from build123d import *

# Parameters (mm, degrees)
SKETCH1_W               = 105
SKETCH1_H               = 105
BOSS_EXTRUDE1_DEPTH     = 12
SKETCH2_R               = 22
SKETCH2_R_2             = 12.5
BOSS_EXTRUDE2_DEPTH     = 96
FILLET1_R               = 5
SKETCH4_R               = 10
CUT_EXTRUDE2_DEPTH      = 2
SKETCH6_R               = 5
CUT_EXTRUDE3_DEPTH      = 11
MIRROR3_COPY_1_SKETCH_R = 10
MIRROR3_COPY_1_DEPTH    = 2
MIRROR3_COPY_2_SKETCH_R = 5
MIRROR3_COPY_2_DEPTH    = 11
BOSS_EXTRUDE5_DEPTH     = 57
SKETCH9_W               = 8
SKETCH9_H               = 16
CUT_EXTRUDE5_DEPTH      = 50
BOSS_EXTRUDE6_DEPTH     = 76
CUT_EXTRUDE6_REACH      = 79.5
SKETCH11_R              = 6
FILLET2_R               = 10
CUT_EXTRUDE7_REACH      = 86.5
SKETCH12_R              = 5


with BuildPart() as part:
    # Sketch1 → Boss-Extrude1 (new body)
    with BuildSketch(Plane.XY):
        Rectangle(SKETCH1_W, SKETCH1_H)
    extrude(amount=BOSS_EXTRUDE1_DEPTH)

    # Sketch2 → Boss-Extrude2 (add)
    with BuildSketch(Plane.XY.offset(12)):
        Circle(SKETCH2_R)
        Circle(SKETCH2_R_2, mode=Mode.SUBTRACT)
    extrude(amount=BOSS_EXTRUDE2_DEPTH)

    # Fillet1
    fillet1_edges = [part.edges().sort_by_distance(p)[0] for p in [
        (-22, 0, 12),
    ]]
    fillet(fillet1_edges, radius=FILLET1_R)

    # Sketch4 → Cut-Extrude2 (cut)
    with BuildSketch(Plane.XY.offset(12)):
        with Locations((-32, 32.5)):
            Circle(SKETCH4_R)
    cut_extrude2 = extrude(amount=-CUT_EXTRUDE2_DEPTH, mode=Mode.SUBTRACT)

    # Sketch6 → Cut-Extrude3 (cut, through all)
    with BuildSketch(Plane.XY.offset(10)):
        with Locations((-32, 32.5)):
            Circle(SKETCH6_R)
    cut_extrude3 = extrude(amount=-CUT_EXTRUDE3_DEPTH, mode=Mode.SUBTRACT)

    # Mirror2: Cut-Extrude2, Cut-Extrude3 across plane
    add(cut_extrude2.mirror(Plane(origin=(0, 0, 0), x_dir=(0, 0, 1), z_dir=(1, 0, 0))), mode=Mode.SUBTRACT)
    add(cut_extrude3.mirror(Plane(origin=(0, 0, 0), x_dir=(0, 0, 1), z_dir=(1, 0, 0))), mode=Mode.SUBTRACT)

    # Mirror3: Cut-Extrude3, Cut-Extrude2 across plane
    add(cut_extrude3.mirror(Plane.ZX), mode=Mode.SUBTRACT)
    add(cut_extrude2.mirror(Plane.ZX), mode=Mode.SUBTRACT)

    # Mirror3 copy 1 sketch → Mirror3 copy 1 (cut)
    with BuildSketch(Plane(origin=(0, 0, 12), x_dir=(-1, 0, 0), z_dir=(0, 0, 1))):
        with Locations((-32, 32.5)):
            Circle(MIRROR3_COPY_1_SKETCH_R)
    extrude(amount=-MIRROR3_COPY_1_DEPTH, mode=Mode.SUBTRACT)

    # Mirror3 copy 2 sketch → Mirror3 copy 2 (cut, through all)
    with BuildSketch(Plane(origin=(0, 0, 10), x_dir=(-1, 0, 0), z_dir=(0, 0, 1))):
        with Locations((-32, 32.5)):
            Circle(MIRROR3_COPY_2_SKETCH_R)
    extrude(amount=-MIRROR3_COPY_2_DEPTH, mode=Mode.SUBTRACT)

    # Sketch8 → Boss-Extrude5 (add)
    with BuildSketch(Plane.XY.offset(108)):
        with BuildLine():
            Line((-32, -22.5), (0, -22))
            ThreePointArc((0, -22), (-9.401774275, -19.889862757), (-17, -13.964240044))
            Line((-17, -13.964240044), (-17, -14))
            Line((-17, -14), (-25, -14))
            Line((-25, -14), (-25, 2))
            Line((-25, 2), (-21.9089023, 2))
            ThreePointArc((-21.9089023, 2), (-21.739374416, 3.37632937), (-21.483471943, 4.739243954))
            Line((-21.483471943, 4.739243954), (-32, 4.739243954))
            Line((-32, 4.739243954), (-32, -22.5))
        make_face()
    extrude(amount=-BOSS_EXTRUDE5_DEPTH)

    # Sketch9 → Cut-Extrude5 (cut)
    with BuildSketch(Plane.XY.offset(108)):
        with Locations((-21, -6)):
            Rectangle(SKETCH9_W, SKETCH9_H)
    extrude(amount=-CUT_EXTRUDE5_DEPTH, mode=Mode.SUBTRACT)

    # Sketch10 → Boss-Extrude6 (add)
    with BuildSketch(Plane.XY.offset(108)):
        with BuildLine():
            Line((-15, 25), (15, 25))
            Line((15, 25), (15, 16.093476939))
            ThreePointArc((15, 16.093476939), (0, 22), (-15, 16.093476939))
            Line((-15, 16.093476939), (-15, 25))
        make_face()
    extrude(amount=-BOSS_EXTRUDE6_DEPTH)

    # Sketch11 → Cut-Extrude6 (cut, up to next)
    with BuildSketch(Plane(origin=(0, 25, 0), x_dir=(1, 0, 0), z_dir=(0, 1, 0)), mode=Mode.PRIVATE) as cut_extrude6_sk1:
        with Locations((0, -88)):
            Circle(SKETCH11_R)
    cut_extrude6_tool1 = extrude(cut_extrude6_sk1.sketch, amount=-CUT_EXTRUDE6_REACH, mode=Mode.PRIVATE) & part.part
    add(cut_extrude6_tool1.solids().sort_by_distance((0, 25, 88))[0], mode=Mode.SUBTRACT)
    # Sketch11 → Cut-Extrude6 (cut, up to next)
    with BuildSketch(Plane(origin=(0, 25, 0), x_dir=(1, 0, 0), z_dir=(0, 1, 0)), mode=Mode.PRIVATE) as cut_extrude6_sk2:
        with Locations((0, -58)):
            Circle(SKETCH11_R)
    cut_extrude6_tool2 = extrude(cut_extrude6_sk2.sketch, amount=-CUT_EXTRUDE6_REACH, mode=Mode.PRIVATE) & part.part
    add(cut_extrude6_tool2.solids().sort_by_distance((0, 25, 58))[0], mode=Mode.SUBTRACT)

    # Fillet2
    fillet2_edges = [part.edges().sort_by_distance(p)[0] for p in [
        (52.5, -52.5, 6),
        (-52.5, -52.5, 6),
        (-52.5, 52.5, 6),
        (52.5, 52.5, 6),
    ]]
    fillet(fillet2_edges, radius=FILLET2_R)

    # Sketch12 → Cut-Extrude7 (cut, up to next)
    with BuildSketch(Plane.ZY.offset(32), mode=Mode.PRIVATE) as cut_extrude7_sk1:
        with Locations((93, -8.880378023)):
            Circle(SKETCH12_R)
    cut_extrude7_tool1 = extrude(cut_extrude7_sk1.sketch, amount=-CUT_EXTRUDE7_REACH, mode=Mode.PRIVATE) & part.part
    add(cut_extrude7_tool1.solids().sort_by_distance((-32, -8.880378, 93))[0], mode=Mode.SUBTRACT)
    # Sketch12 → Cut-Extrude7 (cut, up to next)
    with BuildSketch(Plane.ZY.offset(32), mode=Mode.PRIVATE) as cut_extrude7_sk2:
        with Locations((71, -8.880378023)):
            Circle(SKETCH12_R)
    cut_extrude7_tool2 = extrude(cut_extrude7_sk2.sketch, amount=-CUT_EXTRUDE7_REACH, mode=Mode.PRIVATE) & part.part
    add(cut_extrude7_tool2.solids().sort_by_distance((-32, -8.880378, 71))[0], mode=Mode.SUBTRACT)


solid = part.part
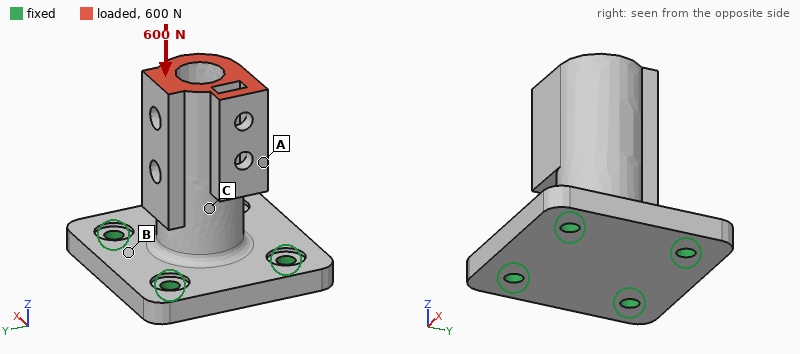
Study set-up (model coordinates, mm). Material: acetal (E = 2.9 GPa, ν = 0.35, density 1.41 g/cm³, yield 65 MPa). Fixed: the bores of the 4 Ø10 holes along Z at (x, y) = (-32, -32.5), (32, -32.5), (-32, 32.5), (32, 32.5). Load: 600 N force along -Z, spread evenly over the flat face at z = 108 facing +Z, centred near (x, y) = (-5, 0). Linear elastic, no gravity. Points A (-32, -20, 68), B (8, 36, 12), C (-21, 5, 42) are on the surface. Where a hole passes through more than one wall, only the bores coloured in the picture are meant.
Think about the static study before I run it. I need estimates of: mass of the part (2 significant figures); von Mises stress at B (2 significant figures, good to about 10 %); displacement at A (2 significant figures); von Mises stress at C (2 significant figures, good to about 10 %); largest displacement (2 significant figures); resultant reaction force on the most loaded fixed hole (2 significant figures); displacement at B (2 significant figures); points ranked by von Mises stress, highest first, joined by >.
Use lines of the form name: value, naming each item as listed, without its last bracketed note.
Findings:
mass of the part: 350 g
von Mises stress at B: 0.59 MPa
displacement at A: 61 µm
von Mises stress at C: 0.88 MPa
largest displacement: 77 µm
resultant reaction force on the most loaded fixed hole: 190 N
displacement at B: 12 µm
points ranked by von Mises stress, highest first, joined by >: C > B > A
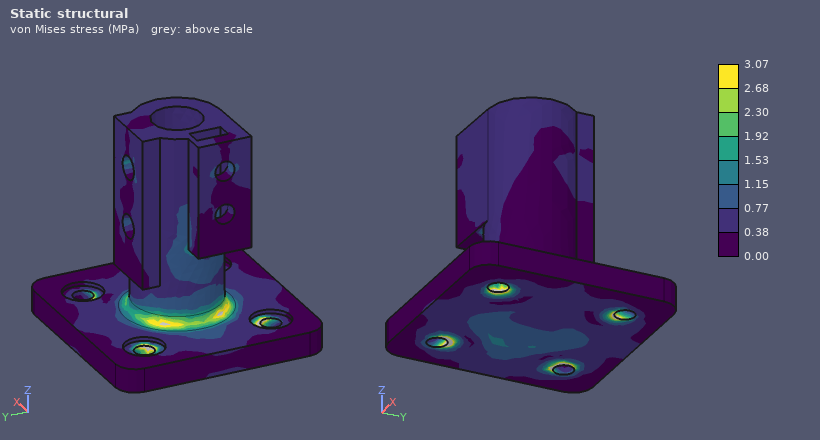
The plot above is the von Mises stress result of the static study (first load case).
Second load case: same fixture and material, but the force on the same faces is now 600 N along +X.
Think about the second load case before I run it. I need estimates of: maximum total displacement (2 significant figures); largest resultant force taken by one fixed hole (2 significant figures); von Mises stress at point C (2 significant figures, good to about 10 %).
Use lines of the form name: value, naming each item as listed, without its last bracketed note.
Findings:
maximum total displacement: 0.89 mm
largest resultant force taken by one fixed hole: 580 N
von Mises stress at point C: 5.1 MPa
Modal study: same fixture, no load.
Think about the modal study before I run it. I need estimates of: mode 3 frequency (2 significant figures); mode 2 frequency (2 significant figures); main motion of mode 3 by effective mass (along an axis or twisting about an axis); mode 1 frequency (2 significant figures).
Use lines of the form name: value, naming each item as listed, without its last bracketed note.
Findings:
mode 3 frequency: 1500 Hz
mode 2 frequency: 570 Hz
main motion of mode 3 by effective mass: along Z
mode 1 frequency: 560 Hz
